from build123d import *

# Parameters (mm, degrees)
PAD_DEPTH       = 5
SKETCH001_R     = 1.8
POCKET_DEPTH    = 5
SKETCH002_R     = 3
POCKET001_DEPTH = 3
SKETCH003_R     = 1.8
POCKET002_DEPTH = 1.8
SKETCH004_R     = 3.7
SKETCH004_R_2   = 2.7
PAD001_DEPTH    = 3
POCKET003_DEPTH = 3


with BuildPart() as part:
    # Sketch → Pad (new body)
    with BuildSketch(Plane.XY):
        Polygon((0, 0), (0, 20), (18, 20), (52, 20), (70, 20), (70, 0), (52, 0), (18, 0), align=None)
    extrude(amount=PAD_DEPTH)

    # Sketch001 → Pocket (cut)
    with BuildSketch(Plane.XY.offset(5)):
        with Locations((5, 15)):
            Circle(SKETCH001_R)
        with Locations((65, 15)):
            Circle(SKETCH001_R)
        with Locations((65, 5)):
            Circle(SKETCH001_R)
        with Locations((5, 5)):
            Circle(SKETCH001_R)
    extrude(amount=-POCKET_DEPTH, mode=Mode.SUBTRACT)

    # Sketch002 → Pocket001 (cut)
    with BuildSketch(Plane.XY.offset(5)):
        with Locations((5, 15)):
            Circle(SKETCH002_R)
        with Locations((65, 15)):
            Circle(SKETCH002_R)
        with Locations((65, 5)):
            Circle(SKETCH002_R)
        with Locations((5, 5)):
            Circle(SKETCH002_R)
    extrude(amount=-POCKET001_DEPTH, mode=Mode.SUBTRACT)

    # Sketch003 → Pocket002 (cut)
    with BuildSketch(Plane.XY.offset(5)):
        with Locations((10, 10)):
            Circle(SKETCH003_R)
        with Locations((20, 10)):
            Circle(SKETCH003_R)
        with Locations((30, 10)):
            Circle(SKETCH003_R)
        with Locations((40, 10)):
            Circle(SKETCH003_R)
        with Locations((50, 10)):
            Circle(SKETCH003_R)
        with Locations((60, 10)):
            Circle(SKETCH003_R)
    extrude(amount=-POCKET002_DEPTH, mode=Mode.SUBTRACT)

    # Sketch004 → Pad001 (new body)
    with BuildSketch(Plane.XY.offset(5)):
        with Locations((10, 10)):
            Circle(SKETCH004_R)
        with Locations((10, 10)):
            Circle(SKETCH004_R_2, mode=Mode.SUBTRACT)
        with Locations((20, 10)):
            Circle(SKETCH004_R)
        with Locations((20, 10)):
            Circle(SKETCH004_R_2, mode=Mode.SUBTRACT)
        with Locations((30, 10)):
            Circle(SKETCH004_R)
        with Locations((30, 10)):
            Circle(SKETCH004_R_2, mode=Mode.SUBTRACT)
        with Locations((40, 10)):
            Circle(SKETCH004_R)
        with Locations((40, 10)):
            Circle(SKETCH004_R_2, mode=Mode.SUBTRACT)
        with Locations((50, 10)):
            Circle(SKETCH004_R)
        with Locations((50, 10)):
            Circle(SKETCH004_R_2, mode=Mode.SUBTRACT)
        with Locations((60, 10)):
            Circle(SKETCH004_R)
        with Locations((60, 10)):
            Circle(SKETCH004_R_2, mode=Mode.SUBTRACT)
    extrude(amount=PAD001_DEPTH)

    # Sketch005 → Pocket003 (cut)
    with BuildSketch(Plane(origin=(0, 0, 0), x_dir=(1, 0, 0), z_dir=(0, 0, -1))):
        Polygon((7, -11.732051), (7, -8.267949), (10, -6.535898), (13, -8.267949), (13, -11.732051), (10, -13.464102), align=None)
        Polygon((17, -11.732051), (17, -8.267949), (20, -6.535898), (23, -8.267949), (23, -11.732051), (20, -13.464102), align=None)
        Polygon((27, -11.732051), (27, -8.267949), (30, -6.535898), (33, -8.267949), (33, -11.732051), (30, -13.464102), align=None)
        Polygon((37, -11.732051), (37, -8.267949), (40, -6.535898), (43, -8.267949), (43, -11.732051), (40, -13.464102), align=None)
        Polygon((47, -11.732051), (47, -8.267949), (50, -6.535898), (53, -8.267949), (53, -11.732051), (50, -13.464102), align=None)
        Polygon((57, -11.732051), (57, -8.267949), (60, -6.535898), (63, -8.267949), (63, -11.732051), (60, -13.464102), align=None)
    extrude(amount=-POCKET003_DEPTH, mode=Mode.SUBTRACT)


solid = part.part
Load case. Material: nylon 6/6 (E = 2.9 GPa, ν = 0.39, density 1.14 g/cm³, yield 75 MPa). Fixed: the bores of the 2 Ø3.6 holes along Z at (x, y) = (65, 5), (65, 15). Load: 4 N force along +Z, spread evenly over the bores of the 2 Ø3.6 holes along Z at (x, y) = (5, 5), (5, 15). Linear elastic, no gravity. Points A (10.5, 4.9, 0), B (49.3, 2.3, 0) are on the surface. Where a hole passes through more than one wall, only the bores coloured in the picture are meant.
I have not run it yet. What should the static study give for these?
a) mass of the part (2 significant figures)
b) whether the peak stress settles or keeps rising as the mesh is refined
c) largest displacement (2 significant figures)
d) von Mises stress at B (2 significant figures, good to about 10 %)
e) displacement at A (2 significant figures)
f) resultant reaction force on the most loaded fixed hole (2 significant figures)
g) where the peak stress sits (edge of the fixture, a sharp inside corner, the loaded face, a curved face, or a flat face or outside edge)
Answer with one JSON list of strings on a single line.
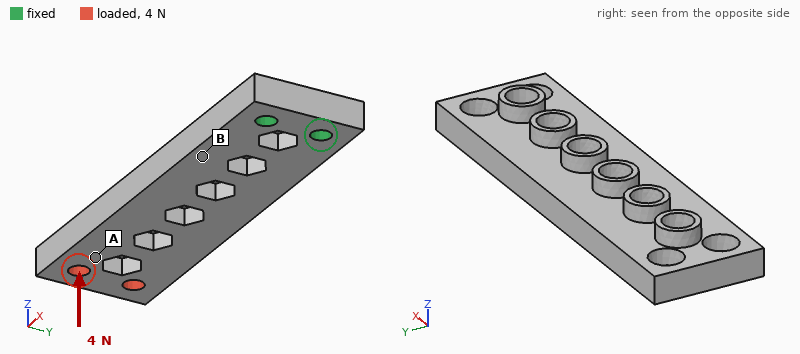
["7.1 g", "keeps rising", "0.82 mm", "2.6 MPa", "0.64 mm", "2.3 N", "edge of the fixture"]
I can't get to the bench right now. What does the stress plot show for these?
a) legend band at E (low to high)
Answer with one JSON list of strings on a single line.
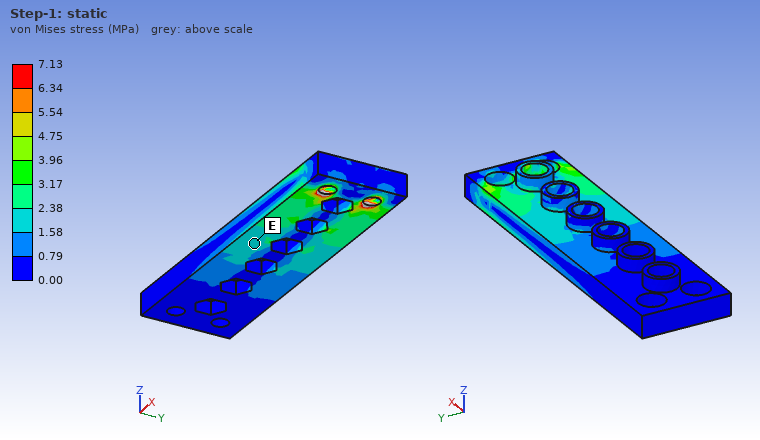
["1.58 to 2.38 MPa"]
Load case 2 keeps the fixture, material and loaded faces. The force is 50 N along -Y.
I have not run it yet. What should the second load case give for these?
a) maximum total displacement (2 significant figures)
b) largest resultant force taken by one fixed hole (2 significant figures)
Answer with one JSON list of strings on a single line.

["0.77 mm", "230 N"]
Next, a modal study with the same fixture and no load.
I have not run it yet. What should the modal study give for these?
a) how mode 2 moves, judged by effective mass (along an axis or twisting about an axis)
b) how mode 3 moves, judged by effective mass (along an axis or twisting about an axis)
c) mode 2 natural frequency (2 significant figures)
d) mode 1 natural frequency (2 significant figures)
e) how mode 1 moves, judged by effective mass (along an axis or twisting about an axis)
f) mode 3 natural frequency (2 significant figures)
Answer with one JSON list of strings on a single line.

["along Y", "twisting about X", "940 Hz", "260 Hz", "along Z", "1600 Hz"]
